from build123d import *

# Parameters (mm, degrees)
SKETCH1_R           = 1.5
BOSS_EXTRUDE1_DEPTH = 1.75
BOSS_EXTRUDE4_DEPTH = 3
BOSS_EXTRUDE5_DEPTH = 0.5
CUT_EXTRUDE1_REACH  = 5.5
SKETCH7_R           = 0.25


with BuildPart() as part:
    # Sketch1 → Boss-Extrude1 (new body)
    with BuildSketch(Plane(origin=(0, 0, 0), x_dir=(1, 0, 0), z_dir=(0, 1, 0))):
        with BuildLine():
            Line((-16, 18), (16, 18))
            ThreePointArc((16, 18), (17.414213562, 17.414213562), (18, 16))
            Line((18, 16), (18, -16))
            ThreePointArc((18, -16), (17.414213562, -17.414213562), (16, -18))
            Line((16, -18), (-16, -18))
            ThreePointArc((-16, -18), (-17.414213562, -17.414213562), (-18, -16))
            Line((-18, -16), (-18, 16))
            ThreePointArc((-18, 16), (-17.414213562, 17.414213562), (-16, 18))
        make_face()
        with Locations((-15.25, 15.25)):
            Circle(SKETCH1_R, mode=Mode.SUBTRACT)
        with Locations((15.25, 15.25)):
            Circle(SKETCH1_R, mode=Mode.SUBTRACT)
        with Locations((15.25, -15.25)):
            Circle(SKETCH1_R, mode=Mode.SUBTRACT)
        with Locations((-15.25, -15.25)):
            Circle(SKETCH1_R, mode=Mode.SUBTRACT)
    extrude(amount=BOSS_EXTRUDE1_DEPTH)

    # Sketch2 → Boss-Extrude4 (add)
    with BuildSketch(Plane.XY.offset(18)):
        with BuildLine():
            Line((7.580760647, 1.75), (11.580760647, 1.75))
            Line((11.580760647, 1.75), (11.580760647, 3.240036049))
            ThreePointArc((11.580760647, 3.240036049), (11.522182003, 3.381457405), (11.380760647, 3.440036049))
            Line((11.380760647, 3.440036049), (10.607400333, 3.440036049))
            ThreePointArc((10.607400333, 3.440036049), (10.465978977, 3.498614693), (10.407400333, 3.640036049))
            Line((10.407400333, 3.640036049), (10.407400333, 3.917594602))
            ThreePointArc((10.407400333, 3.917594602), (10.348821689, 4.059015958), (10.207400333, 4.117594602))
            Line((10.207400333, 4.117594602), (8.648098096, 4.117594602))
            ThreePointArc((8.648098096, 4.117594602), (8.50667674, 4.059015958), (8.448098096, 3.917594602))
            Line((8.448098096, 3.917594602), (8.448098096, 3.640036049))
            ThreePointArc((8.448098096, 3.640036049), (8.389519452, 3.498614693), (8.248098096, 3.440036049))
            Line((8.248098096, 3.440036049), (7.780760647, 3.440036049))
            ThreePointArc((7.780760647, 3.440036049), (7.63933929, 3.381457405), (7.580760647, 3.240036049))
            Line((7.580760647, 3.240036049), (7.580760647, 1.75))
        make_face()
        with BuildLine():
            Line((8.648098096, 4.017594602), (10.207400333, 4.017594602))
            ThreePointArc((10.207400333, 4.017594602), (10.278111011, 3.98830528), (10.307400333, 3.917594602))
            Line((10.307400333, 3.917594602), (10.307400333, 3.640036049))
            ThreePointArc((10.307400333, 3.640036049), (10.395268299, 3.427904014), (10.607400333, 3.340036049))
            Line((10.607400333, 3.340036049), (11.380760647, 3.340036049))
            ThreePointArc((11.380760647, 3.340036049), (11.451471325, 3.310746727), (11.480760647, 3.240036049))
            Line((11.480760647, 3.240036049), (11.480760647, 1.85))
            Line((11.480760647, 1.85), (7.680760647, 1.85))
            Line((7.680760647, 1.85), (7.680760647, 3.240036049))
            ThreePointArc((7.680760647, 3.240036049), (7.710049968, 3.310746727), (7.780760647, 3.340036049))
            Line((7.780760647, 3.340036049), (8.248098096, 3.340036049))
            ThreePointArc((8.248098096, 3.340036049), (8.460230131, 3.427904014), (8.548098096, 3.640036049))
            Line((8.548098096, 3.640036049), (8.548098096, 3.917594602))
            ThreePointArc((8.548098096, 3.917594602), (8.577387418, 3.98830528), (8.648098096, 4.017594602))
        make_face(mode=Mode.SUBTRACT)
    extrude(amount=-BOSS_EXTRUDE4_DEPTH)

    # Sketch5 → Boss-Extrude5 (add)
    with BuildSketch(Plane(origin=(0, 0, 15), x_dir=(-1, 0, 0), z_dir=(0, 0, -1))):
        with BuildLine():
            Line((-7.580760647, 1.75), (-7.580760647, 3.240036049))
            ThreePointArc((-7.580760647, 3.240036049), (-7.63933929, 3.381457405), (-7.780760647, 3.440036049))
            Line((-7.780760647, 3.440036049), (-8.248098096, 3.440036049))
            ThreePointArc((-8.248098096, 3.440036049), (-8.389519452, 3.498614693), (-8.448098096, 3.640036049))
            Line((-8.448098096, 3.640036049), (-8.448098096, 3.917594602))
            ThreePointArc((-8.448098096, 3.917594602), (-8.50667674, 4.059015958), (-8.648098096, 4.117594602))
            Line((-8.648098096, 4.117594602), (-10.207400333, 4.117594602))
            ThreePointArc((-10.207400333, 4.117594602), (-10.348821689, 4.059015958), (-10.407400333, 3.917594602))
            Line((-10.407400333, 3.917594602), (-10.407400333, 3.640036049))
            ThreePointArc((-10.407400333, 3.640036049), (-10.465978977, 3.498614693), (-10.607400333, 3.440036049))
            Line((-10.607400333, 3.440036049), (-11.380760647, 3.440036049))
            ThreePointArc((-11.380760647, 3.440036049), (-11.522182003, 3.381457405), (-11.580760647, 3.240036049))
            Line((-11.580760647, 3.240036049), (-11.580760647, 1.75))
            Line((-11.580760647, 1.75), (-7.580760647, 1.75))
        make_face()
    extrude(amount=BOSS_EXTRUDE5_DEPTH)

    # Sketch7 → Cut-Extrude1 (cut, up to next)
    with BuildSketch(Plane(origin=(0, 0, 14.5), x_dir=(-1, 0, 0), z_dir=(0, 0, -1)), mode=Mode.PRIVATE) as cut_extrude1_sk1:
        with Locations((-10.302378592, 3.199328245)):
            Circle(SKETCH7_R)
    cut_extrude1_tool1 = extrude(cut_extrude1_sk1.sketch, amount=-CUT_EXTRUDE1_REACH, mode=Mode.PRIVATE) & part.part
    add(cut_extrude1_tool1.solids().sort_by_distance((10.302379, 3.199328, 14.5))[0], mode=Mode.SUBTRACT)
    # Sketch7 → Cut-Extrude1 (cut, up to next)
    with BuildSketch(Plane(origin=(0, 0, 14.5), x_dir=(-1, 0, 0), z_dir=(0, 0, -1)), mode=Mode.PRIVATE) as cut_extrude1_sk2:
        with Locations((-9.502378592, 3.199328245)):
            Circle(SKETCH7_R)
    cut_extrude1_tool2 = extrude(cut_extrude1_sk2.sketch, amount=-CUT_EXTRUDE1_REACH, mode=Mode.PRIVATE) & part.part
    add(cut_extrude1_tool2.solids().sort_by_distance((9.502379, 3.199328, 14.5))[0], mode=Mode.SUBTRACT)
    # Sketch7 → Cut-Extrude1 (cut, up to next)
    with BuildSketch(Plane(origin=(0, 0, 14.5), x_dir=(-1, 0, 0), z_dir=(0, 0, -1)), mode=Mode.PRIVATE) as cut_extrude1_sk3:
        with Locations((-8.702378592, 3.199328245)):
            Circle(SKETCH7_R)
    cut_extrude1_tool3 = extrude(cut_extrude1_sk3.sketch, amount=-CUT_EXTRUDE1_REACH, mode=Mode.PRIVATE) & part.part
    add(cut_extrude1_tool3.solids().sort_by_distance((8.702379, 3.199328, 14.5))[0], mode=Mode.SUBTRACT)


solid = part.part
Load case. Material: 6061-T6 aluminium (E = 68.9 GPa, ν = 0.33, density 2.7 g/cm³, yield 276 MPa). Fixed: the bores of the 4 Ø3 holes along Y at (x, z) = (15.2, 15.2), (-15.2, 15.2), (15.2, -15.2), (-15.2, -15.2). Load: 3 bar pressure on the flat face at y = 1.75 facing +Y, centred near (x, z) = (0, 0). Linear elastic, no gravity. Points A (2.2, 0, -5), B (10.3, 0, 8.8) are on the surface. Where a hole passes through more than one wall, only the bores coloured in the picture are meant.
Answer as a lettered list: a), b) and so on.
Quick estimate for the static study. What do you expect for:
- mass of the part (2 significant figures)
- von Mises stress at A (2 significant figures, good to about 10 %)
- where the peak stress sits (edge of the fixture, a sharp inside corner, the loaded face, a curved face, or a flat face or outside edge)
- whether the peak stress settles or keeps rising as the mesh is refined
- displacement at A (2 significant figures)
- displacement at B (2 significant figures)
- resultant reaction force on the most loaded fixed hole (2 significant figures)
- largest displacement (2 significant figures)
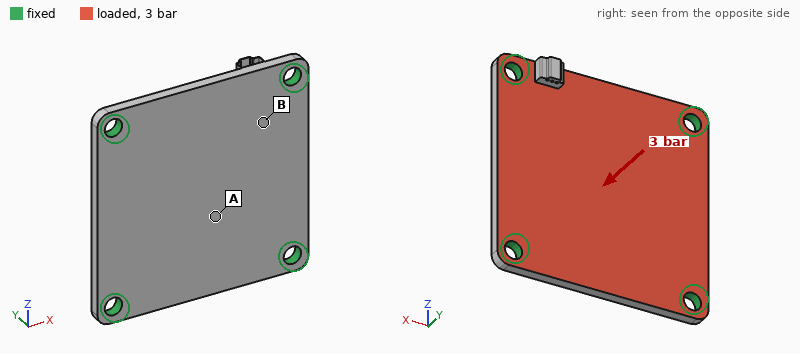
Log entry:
a) 6.0 g
b) 25 MPa
c) edge of the fixture
d) keeps rising
e) 45 µm
f) 22 µm
g) 95 N
h) 49 µm
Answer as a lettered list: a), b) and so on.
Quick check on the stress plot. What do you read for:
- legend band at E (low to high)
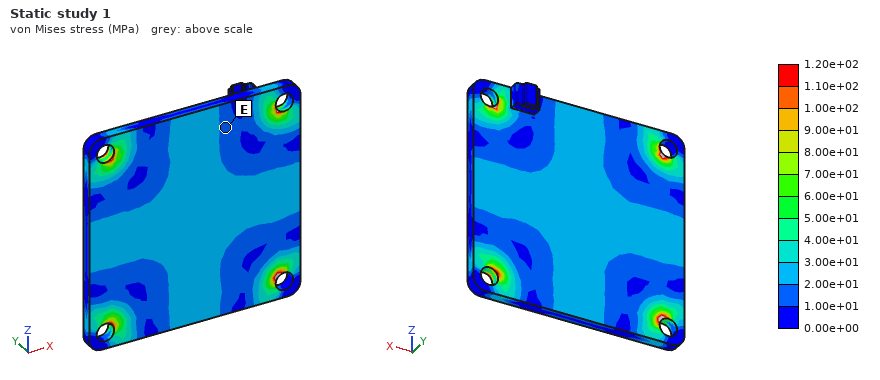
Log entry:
a) 1.00e+01 to 2.00e+01 MPa
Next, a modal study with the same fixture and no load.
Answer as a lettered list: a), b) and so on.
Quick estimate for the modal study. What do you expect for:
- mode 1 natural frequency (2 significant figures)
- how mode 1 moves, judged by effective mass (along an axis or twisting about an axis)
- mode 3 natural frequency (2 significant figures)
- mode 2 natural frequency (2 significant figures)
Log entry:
a) 7000 Hz
b) along Y
c) 12 kHz
d) 12 kHz
